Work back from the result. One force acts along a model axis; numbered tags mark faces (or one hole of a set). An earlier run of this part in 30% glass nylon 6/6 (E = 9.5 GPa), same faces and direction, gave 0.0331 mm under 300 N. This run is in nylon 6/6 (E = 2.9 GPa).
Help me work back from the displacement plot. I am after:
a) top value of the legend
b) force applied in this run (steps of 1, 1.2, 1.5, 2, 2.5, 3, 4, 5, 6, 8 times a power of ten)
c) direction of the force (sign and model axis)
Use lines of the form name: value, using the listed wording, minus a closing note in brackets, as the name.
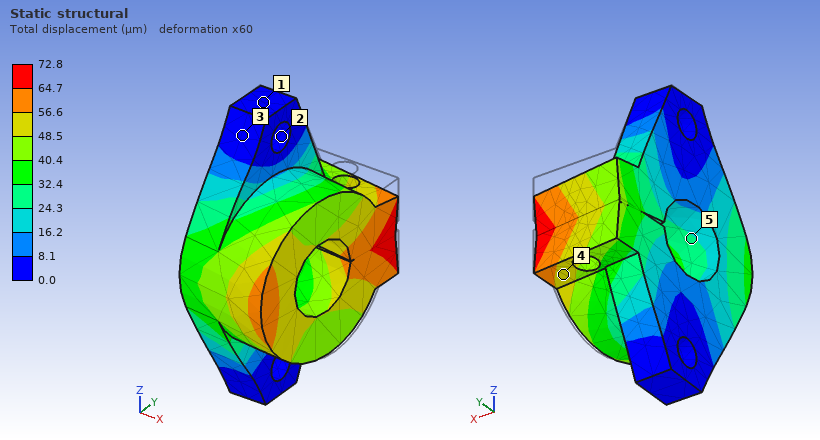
top value of the legend: 72.8 µm
force applied in this run: 200 N
direction of the force: -Y
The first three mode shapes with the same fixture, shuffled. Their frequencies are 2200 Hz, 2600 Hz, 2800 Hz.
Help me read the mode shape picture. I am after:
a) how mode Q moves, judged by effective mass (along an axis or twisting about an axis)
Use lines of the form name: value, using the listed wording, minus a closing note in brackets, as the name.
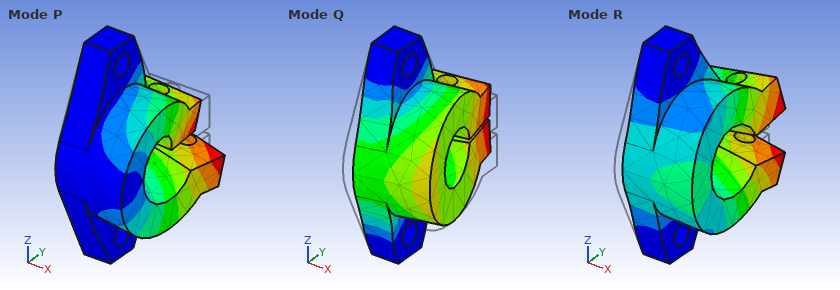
how mode Q moves, judged by effective mass: along Y
